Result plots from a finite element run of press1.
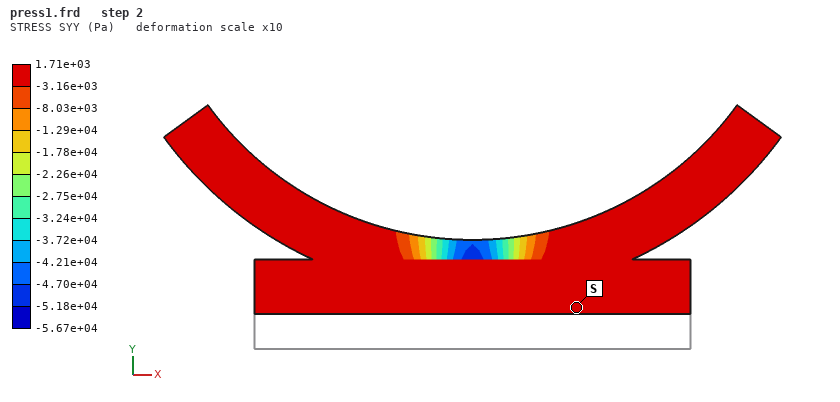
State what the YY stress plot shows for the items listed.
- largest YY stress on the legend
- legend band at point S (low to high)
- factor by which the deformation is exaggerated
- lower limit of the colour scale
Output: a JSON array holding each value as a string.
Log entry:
["1.71e+03 Pa", "-3.16e+03 to 1.71e+03 Pa", "10", "-5.67e+04 Pa"]
